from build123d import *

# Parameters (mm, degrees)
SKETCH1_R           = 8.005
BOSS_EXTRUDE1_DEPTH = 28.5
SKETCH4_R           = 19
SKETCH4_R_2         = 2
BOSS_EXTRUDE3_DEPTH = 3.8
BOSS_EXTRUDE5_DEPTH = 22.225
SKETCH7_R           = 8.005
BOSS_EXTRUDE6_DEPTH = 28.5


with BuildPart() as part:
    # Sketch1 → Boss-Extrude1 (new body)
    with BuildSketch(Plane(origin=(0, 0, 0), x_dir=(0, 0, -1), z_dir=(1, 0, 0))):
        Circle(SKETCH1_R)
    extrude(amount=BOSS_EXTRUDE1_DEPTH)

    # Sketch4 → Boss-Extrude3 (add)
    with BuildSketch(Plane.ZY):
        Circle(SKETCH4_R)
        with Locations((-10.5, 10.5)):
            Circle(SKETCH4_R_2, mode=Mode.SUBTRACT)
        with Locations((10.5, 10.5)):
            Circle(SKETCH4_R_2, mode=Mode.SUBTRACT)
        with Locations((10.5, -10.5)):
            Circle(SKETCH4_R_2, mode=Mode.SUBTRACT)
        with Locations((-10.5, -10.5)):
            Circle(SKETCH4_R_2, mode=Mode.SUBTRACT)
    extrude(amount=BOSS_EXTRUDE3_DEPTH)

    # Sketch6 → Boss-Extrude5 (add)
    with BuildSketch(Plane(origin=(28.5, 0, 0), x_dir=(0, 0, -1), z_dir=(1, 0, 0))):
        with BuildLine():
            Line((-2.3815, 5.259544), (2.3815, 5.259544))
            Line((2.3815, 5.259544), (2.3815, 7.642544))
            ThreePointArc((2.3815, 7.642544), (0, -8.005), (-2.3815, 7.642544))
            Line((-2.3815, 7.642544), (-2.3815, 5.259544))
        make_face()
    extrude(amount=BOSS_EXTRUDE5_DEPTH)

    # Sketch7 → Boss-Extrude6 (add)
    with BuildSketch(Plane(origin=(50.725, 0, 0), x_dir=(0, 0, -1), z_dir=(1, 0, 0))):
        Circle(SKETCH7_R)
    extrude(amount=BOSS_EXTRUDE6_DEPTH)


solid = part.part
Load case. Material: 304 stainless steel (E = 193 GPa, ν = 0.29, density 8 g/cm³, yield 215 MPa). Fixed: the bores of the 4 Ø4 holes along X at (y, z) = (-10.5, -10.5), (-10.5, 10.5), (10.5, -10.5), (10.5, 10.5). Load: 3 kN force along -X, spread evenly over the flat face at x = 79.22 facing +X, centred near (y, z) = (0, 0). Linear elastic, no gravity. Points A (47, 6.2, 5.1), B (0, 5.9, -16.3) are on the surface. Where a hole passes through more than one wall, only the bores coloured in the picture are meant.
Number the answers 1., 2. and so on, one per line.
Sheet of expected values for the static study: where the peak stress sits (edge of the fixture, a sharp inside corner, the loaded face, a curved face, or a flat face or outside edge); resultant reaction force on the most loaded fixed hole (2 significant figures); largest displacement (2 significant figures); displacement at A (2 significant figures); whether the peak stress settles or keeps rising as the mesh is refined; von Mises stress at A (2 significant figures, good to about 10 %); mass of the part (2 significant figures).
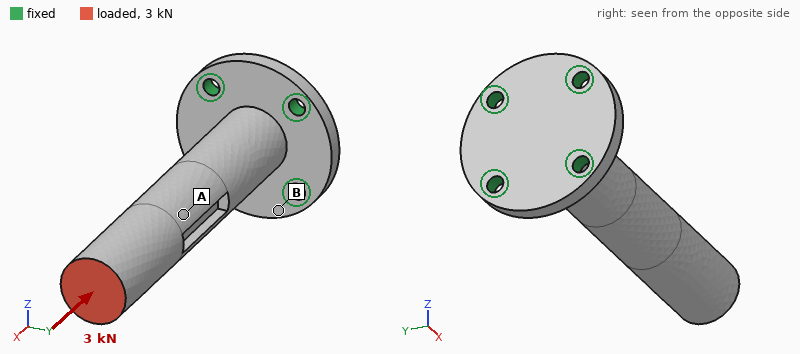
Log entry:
1. edge of the fixture
2. 780 N
3. 12 µm
4. 8.6 µm
5. keeps rising
6. 19 MPa
7. 160 g
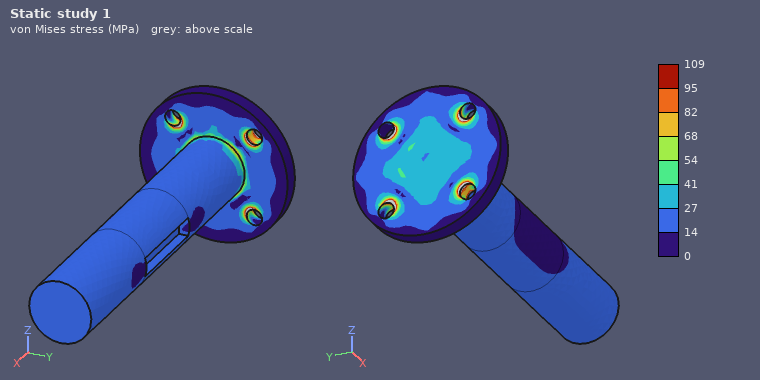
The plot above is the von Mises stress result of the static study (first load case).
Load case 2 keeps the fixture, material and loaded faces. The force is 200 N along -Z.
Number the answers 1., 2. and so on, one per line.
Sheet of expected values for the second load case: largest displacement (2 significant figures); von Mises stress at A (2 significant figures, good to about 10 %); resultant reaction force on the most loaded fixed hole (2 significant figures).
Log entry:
1. 85 µm
2. 11 MPa
3. 450 N
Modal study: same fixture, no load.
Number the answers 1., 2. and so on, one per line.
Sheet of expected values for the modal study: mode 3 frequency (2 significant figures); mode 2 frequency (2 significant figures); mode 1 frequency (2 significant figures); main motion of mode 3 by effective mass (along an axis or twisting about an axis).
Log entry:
1. 7800 Hz
2. 1300 Hz
3. 1300 Hz
4. along Y
